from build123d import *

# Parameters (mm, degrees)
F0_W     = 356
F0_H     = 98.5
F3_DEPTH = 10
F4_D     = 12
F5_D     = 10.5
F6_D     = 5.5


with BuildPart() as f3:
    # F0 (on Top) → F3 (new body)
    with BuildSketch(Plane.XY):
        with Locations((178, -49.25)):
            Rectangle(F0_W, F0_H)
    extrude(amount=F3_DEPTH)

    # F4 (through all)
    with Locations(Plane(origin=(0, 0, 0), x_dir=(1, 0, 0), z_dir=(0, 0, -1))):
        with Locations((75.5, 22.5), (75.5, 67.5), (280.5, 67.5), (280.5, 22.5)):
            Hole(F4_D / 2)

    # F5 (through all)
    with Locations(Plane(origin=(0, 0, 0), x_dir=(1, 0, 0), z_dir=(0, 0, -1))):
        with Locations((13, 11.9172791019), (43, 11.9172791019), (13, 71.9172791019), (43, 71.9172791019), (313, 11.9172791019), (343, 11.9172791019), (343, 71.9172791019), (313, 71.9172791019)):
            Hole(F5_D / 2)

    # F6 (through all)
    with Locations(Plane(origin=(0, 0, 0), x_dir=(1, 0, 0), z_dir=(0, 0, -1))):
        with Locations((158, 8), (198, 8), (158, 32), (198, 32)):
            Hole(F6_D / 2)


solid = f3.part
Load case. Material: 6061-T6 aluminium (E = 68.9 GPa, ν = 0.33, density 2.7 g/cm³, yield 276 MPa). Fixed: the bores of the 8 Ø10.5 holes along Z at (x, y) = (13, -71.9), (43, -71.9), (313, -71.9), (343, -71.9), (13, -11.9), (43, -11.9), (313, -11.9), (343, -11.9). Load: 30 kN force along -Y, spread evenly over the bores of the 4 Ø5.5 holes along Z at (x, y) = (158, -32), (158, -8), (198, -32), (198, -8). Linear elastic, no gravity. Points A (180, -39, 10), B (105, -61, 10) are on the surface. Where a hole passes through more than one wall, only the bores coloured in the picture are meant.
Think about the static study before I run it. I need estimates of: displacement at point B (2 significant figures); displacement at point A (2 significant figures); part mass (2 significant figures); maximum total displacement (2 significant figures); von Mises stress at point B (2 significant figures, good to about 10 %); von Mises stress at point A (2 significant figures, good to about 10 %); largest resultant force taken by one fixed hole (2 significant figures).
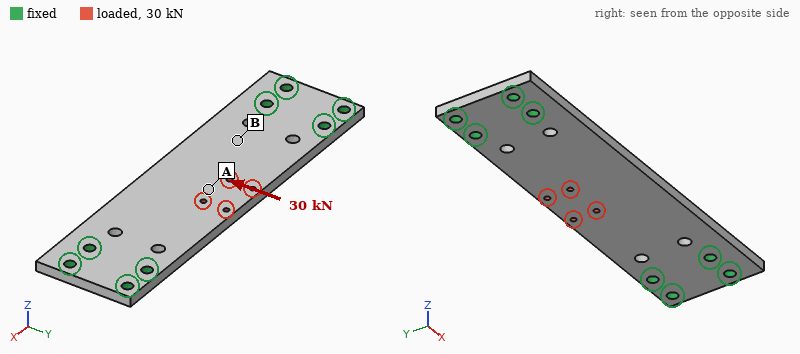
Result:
0.080 mm
0.15 mm
910 g
0.16 mm
38 MPa
16 MPa
14 kN
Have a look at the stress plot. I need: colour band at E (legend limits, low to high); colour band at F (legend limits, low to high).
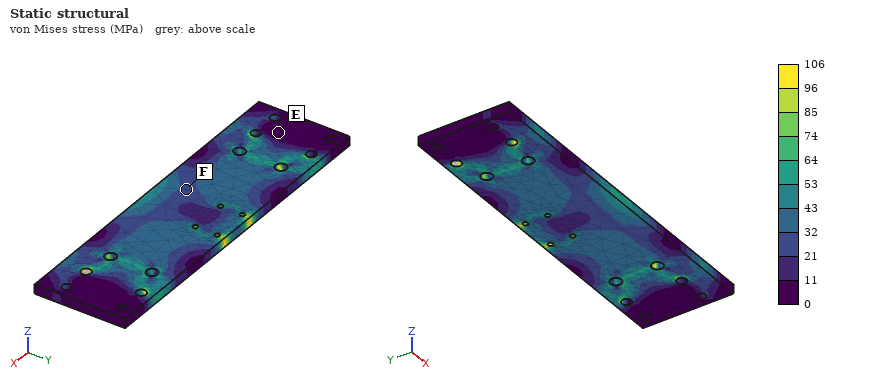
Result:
0 to 11 MPa
21 to 32 MPa
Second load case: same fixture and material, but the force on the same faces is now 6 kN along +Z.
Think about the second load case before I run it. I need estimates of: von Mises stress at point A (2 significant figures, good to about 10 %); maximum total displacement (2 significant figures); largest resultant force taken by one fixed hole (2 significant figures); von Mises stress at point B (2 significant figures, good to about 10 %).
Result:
89 MPa
1.6 mm
3.2 kN
39 MPa
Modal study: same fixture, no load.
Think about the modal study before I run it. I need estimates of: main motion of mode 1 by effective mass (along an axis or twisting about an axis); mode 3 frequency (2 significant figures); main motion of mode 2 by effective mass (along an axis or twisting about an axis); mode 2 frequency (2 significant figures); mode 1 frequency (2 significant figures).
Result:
along Z
2000 Hz
twisting about X
1400 Hz
710 Hz
